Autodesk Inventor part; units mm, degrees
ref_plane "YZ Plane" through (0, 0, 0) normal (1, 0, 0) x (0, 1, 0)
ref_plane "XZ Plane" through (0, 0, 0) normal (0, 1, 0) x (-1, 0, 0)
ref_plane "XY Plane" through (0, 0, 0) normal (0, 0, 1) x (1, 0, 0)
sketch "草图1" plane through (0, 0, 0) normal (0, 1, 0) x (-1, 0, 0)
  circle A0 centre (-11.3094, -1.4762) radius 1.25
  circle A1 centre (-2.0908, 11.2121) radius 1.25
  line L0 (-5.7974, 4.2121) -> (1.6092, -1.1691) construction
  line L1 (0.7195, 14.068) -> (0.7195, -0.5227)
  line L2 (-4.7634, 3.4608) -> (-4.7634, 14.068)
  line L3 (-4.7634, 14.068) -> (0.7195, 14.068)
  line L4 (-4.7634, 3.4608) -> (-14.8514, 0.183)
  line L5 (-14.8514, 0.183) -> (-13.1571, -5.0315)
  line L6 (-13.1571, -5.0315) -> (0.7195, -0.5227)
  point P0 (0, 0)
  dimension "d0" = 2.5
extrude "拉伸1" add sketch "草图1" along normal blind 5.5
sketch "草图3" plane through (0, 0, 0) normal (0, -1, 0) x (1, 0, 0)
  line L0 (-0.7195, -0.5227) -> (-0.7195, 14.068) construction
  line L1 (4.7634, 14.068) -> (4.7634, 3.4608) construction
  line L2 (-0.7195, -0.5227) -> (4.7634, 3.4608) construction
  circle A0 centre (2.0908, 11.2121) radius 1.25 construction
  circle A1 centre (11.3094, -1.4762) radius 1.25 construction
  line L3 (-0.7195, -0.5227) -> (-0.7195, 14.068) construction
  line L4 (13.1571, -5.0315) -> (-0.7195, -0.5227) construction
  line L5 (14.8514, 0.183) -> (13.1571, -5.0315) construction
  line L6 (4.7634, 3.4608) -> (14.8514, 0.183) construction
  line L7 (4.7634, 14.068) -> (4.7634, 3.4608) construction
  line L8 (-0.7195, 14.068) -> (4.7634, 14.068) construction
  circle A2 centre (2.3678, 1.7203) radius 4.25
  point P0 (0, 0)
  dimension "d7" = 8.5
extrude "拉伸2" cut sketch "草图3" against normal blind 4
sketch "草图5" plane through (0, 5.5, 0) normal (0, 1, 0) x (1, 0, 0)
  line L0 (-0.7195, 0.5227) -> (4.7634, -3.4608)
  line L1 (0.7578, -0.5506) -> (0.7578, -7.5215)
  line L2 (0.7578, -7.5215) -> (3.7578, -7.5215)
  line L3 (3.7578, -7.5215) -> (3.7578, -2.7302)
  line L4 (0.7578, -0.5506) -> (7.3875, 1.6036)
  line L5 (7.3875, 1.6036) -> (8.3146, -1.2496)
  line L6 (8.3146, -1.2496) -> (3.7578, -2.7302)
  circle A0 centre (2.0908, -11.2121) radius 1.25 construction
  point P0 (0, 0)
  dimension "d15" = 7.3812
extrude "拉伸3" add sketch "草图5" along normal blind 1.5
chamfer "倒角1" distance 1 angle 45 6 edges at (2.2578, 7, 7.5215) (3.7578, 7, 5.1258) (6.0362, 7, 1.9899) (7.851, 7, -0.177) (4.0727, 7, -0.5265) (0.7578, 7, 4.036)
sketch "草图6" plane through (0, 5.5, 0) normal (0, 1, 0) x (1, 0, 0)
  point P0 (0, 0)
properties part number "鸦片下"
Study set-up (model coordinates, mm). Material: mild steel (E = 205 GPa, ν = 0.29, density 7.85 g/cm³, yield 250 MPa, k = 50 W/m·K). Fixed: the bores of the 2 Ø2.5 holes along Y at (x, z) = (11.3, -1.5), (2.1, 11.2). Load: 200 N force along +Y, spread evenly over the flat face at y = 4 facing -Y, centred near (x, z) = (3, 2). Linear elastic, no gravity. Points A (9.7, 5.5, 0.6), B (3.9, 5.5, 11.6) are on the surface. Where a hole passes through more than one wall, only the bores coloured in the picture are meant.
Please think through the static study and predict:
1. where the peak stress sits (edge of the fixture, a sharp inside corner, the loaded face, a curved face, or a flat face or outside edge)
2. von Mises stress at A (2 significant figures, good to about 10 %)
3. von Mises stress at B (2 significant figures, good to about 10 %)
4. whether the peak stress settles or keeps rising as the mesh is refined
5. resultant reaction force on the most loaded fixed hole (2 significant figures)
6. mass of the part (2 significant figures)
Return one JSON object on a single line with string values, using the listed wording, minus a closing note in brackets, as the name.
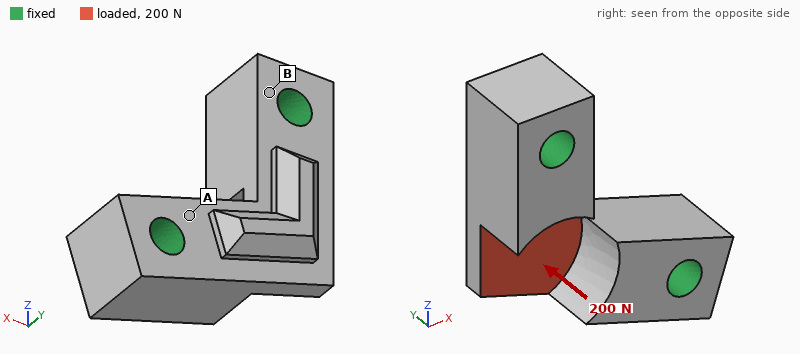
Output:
{"where the peak stress sits": "a sharp inside corner", "von Mises stress at A": "18 MPa", "von Mises stress at B": "6.5 MPa", "whether the peak stress settles or keeps rising as the mesh is refined": "keeps rising", "resultant reaction force on the most loaded fixed hole": "110 N", "mass of the part": "4.4 g"}
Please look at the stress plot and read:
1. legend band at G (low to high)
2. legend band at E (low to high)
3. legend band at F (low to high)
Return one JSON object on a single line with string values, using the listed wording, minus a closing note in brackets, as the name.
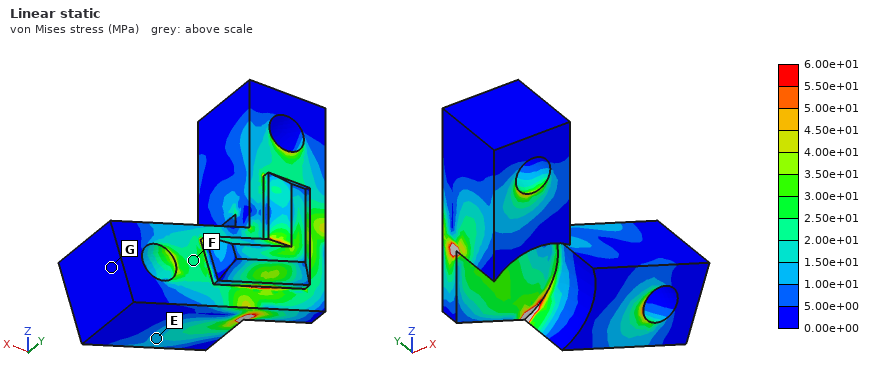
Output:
{"legend band at G": "0.00e+00 to 5.00e+00 MPa", "legend band at E": "1.00e+01 to 1.50e+01 MPa", "legend band at F": "2.00e+01 to 2.50e+01 MPa"}
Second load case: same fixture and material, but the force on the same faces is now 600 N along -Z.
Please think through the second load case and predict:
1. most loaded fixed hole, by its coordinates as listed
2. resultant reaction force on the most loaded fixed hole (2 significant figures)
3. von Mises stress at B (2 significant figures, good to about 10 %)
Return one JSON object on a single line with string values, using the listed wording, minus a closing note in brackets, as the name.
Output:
{"most loaded fixed hole, by its coordinates as listed": "(2.1, 11.2)", "resultant reaction force on the most loaded fixed hole": "460 N", "von Mises stress at B": "16 MPa"}
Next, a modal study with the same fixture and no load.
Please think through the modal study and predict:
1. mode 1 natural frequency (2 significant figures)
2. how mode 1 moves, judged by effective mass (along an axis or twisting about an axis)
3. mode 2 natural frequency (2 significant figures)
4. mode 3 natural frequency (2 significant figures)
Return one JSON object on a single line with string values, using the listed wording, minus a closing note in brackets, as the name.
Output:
{"mode 1 natural frequency": "48 kHz", "how mode 1 moves, judged by effective mass": "along Y", "mode 2 natural frequency": "89 kHz", "mode 3 natural frequency": "94 kHz"}
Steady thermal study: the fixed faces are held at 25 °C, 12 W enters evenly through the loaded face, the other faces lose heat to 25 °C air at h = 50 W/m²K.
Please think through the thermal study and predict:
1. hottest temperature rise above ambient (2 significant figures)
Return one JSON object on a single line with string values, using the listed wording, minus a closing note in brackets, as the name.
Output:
{"hottest temperature rise above ambient": "64 K"}
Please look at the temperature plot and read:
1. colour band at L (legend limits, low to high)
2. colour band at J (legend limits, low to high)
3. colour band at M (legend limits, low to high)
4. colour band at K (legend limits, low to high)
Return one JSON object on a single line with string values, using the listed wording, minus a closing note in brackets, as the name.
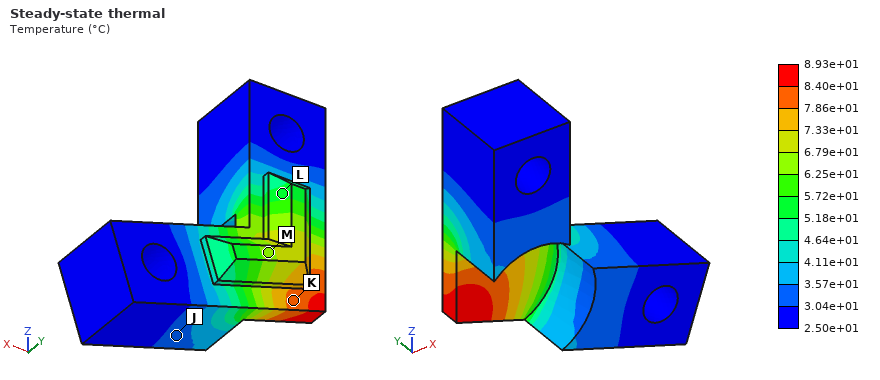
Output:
{"colour band at L": "5.18e+01 to 5.72e+01 °C", "colour band at J": "3.04e+01 to 3.57e+01 °C", "colour band at M": "6.25e+01 to 6.79e+01 °C", "colour band at K": "7.86e+01 to 8.40e+01 °C"}
